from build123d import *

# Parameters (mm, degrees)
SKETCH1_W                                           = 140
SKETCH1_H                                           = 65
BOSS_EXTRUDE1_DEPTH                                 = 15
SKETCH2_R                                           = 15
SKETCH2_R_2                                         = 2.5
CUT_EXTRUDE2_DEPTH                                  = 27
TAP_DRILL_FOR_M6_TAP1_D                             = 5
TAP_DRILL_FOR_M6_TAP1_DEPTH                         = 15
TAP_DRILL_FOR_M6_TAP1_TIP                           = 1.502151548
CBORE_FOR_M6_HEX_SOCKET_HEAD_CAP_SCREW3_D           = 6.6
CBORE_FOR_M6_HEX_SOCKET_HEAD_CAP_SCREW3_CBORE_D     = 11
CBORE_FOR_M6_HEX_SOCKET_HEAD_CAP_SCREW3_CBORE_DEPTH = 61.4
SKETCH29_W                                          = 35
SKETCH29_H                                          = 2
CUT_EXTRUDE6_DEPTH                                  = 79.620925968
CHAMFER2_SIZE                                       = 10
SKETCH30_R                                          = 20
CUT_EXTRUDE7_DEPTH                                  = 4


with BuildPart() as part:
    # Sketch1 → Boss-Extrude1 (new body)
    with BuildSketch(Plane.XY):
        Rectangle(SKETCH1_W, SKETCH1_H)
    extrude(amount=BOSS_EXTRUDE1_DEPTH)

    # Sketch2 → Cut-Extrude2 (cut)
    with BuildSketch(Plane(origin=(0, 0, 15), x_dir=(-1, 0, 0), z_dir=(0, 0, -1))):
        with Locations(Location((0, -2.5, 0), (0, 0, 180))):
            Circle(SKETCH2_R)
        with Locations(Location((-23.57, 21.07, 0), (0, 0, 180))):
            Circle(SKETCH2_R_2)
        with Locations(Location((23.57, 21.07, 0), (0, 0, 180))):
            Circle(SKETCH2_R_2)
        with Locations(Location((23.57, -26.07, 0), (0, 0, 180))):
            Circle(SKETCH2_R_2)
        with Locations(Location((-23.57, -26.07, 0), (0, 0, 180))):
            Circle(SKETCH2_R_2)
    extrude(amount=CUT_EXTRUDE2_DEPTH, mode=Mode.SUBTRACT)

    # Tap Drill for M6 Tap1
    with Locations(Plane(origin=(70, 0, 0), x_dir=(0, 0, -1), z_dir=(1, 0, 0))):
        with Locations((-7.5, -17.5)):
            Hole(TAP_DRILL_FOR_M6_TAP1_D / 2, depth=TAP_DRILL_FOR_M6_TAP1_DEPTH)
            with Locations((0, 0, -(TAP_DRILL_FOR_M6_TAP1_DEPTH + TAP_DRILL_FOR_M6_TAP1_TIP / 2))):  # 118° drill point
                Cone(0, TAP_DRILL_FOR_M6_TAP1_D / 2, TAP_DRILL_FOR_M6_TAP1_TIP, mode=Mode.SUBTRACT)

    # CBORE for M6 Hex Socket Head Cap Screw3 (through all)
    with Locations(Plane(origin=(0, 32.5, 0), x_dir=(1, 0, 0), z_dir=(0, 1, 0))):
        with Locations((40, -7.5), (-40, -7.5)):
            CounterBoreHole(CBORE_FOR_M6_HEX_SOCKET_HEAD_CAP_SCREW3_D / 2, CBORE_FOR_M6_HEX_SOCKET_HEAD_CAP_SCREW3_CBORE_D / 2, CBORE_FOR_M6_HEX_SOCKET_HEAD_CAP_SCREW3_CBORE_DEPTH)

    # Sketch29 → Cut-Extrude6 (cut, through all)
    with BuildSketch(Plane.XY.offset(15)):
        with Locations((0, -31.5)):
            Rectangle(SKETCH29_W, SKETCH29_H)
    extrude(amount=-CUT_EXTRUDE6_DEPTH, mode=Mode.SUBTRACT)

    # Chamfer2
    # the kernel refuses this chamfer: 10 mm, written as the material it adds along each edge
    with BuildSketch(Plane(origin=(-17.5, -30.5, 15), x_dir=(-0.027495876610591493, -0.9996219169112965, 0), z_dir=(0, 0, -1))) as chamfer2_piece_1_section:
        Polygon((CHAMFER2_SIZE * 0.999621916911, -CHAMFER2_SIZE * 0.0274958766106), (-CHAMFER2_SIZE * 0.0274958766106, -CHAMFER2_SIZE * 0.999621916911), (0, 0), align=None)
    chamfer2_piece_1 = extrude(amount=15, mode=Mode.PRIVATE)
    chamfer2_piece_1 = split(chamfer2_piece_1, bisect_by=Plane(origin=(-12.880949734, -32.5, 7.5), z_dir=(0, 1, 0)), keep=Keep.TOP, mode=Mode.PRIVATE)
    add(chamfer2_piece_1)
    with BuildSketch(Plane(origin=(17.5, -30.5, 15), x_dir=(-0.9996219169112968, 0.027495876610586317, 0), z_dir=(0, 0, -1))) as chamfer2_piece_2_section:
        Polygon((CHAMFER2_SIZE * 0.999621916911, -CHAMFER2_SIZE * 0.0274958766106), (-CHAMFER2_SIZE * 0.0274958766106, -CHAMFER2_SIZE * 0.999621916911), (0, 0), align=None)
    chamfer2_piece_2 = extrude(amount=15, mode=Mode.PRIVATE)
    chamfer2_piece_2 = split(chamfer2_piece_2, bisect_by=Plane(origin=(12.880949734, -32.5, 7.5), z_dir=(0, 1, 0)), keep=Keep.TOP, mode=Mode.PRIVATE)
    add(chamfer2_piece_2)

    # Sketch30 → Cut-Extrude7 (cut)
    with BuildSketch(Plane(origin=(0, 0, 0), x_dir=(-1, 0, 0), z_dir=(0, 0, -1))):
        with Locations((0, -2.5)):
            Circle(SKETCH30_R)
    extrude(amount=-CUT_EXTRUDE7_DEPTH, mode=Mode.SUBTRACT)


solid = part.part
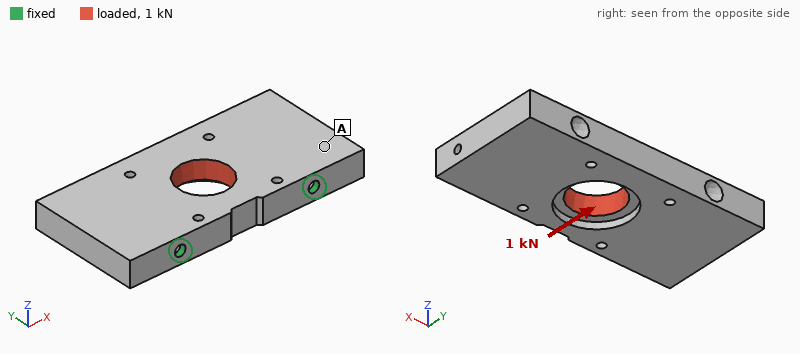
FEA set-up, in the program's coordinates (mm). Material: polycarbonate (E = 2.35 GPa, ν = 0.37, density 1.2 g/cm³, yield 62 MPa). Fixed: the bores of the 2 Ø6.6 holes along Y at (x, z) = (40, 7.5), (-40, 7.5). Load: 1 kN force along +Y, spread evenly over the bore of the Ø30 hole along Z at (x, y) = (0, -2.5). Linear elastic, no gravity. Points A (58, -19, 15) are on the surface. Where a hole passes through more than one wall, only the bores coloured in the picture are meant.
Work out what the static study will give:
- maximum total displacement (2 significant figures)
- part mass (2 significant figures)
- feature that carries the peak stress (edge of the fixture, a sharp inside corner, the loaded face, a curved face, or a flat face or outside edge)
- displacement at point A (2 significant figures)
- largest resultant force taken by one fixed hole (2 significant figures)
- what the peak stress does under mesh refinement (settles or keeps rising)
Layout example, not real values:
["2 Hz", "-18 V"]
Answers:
["0.33 mm", "130 g", "edge of the fixture", "0.080 mm", "530 N", "keeps rising"]
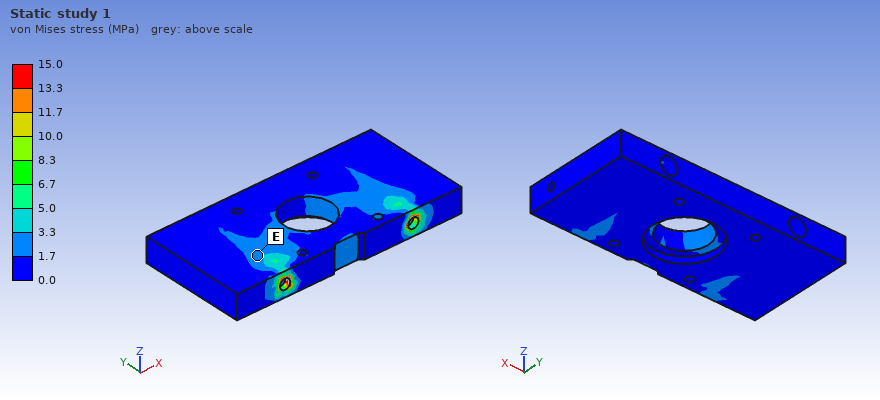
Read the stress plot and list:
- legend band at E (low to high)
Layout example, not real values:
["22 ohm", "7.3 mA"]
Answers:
["1.7 to 3.3 MPa"]
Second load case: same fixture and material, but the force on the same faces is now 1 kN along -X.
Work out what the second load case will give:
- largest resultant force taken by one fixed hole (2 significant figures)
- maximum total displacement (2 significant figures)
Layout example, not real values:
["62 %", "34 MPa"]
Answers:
["610 N", "0.18 mm"]
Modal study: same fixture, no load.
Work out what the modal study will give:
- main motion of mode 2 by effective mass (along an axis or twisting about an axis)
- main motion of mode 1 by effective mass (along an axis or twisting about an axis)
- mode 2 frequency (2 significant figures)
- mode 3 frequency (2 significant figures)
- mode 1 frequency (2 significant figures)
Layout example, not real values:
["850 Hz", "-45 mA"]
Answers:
["twisting about Y", "along Z", "570 Hz", "1100 Hz", "250 Hz"]
